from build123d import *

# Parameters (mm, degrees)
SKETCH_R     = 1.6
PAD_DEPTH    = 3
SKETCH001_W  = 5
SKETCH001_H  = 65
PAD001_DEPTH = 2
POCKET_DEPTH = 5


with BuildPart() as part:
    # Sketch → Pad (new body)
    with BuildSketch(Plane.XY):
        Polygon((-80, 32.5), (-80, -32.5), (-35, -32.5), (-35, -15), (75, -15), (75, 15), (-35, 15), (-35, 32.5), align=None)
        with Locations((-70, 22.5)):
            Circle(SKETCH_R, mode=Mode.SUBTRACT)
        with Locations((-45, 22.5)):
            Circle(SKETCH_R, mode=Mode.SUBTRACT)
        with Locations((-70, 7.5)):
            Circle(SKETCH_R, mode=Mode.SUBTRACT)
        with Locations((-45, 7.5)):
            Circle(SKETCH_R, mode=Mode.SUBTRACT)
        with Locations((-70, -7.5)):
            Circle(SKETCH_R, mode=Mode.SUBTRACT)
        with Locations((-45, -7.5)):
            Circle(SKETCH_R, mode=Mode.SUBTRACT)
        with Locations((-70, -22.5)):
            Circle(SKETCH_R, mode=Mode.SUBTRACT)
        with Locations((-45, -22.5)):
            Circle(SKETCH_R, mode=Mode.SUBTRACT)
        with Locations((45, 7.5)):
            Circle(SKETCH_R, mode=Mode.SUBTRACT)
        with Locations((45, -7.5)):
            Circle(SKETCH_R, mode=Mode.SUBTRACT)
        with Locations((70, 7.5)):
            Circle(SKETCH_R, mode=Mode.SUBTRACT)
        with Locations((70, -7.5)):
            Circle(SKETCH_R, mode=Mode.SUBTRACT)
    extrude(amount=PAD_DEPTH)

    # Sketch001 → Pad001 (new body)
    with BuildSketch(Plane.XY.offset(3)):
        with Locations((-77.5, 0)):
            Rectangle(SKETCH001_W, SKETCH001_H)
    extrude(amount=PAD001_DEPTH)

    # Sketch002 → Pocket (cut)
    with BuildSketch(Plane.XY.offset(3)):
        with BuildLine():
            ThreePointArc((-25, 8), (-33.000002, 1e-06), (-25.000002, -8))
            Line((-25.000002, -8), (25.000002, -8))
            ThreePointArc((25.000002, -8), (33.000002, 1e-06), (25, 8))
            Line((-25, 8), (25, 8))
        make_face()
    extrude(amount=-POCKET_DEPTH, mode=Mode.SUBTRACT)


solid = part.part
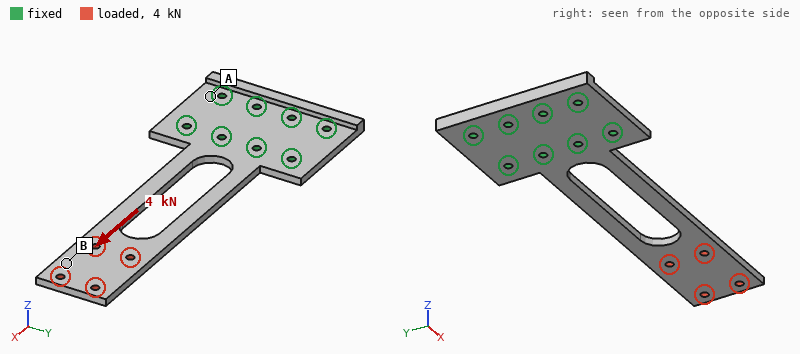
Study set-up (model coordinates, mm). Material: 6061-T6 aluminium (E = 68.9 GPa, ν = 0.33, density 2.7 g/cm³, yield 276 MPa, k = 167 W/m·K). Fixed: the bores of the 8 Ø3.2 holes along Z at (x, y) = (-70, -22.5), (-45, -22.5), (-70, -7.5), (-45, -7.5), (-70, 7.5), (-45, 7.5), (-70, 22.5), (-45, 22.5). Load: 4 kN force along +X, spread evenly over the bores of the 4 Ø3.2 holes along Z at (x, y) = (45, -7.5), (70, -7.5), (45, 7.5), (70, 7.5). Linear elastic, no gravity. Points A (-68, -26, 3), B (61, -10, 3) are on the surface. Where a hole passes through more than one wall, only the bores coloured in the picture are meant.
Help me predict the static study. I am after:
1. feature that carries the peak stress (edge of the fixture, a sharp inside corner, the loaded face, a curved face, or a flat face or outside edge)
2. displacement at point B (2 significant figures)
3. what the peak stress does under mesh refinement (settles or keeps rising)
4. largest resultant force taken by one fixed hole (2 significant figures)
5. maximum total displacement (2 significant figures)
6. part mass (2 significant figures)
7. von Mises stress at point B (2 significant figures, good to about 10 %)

a sharp inside corner
0.12 mm
keeps rising
1.3 kN
0.13 mm
43 g
25 MPa
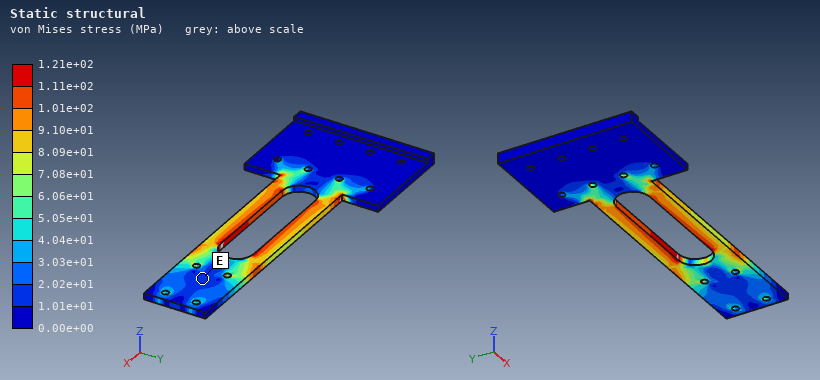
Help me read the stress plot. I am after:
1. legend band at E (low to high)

1.01e+01 to 2.02e+01 MPa
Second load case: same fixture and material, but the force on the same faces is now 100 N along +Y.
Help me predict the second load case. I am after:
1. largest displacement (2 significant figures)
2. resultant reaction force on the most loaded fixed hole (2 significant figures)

0.29 mm
170 N
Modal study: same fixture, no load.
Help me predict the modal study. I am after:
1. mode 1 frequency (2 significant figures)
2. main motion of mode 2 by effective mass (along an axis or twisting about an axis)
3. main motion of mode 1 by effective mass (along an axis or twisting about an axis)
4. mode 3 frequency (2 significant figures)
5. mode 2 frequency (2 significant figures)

140 Hz
along Y
along Z
960 Hz
890 Hz
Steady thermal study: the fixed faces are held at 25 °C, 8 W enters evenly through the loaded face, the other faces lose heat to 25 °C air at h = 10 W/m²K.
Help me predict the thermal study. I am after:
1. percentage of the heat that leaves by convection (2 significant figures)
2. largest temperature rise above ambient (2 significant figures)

33 %
68 K
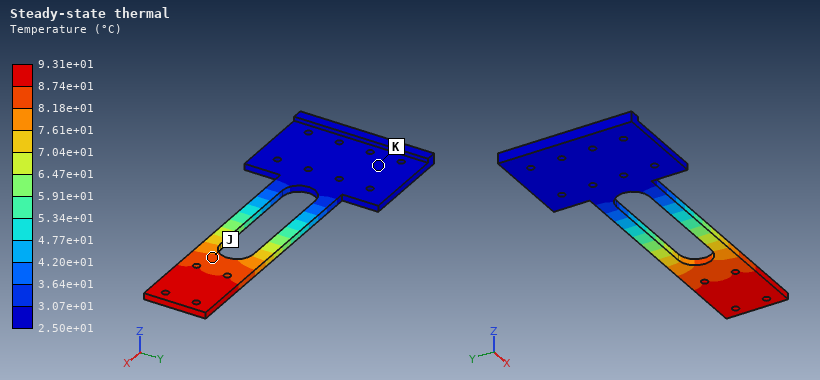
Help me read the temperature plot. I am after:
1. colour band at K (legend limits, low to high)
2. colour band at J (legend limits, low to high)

2.50e+01 to 3.07e+01 °C
8.18e+01 to 8.74e+01 °C
